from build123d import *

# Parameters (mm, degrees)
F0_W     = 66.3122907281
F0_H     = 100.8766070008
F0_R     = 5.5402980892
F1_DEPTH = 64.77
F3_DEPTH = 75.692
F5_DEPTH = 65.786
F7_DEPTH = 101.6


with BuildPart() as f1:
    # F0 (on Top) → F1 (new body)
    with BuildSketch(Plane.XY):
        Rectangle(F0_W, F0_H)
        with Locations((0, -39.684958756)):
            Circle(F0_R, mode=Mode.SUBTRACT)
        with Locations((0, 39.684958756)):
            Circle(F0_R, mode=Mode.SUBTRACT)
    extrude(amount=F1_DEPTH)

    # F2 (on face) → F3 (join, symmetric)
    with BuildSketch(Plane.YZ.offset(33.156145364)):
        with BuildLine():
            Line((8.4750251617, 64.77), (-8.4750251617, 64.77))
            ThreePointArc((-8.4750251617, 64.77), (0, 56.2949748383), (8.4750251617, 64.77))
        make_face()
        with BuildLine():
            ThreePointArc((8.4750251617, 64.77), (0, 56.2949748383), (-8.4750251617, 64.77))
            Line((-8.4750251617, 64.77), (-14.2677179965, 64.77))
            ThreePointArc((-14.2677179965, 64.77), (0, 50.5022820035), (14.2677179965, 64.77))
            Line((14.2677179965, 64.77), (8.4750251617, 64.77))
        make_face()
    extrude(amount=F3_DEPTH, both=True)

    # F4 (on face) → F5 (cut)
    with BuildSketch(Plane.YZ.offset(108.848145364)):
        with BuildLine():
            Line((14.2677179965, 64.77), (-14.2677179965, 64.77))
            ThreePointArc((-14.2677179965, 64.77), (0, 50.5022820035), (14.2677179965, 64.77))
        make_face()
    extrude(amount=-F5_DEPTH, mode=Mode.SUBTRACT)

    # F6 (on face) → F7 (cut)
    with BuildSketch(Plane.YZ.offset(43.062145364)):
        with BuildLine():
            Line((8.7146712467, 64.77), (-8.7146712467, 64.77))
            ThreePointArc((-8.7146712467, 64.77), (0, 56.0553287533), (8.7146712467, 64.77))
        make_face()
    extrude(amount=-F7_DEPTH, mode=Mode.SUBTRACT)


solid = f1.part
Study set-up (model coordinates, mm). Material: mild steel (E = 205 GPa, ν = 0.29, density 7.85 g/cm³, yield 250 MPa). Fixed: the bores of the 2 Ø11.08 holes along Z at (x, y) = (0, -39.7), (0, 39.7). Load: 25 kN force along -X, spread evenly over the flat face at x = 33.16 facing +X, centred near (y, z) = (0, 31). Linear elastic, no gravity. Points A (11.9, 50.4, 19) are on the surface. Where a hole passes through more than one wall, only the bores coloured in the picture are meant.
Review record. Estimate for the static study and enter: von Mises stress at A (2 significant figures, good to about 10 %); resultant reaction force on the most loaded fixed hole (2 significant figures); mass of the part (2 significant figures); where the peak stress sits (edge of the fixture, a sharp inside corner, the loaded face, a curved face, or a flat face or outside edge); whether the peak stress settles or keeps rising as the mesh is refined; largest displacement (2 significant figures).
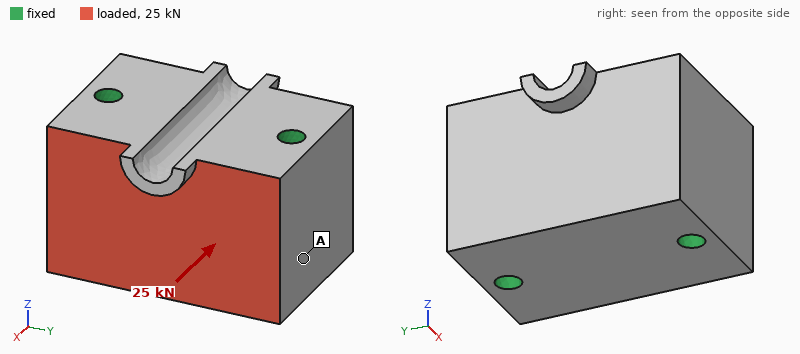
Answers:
2.5 MPa
13 kN
3.3 kg
edge of the fixture
keeps rising
1.5 µm
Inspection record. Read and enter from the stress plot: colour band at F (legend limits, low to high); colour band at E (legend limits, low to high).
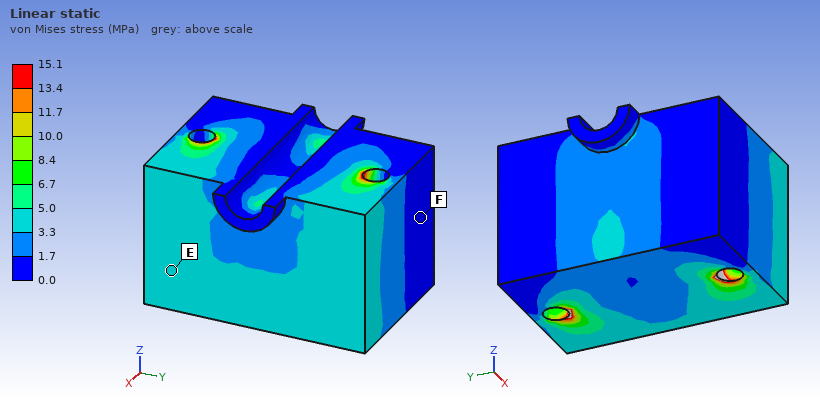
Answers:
0.0 to 1.7 MPa
3.3 to 5.0 MPa
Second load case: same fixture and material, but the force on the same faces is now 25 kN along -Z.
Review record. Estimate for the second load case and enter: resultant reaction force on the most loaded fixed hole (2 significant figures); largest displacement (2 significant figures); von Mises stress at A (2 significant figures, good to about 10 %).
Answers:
13 kN
5.1 µm
11 MPa
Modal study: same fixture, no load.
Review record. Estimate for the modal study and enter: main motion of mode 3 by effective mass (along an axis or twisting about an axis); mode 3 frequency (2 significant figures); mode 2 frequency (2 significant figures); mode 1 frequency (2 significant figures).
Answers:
along X
15 kHz
14 kHz
14 kHz
